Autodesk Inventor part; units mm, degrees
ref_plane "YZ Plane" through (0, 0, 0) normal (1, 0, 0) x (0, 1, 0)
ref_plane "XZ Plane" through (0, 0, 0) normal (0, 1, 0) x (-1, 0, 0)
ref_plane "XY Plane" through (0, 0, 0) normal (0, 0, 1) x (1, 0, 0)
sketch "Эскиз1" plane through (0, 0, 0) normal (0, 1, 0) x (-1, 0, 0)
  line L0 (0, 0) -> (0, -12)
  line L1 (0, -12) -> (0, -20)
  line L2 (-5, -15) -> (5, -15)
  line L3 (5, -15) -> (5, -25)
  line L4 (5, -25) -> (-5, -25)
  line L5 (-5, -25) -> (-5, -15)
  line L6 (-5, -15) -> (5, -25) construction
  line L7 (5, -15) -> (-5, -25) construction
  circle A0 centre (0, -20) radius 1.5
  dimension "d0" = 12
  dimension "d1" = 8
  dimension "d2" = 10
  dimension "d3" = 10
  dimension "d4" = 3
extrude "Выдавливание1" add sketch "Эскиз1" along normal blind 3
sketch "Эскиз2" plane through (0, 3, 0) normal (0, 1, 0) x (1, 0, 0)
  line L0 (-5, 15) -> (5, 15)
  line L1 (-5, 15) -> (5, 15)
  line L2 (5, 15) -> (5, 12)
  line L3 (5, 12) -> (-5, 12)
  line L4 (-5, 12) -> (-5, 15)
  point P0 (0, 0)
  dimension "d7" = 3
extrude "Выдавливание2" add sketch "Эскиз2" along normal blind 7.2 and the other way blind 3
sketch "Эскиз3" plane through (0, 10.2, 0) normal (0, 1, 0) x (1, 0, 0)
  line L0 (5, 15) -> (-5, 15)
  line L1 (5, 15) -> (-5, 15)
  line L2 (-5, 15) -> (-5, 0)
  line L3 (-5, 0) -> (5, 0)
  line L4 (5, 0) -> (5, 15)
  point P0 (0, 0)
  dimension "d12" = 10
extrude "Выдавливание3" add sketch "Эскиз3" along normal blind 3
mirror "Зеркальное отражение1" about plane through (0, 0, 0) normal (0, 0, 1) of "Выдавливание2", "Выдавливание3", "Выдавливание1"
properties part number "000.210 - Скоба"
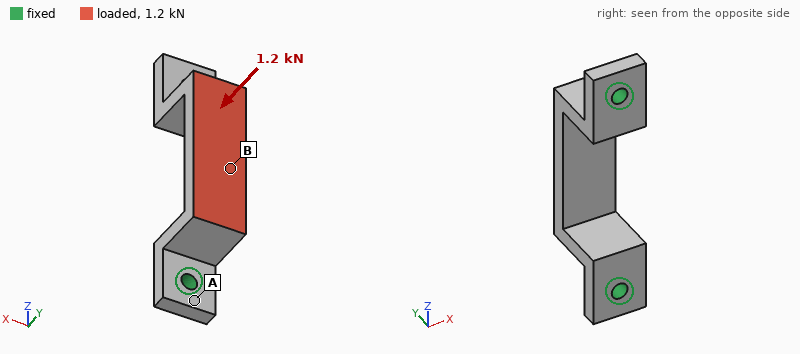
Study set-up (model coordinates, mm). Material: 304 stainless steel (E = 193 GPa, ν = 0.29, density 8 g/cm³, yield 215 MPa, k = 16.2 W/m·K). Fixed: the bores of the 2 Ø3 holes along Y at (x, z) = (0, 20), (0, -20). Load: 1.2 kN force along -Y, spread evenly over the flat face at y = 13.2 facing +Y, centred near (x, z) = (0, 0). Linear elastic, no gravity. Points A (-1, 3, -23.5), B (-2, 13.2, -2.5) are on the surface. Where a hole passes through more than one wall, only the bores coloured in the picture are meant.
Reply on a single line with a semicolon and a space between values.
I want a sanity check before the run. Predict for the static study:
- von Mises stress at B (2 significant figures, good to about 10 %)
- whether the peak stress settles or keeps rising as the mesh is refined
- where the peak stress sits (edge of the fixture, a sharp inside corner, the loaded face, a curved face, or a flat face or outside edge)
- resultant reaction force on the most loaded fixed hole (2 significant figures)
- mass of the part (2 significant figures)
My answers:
92 MPa; keeps rising; edge of the fixture; 710 N; 17 g
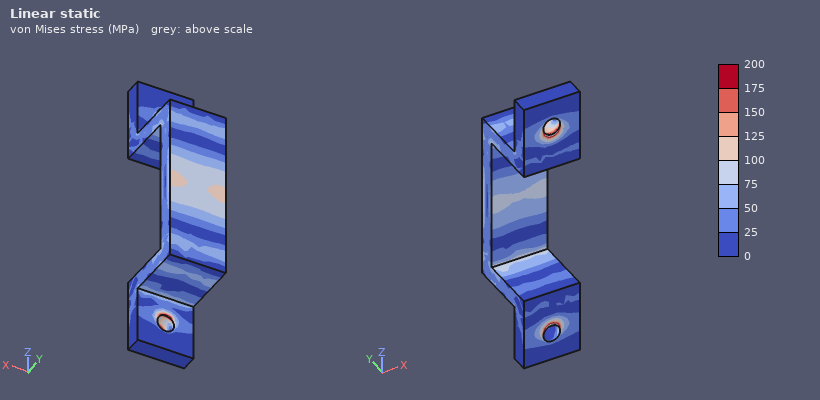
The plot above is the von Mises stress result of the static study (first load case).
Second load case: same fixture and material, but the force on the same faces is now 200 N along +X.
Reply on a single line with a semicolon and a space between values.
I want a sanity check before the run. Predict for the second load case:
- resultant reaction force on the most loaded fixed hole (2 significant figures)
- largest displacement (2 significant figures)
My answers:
100 N; 15 µm
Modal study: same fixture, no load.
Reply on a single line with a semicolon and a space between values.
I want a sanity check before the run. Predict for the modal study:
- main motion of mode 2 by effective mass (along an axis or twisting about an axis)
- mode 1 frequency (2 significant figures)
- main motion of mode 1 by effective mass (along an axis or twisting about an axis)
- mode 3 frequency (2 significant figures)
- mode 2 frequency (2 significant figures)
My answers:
along Z; 7400 Hz; along X; 13 kHz; 9600 Hz
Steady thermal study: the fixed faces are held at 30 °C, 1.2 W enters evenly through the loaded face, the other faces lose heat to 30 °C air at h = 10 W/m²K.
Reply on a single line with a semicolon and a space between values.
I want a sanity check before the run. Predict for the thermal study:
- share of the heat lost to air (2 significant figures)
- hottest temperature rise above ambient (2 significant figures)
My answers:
13 %; 22 K
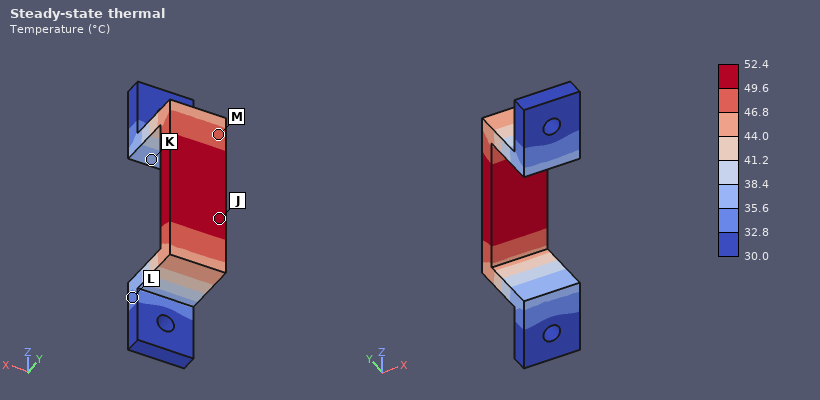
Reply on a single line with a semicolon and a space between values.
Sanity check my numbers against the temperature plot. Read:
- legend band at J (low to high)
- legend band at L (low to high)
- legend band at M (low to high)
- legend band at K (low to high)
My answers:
49.6 to 52.4 °C; 32.8 to 35.6 °C; 46.8 to 49.6 °C; 35.6 to 38.4 °C
